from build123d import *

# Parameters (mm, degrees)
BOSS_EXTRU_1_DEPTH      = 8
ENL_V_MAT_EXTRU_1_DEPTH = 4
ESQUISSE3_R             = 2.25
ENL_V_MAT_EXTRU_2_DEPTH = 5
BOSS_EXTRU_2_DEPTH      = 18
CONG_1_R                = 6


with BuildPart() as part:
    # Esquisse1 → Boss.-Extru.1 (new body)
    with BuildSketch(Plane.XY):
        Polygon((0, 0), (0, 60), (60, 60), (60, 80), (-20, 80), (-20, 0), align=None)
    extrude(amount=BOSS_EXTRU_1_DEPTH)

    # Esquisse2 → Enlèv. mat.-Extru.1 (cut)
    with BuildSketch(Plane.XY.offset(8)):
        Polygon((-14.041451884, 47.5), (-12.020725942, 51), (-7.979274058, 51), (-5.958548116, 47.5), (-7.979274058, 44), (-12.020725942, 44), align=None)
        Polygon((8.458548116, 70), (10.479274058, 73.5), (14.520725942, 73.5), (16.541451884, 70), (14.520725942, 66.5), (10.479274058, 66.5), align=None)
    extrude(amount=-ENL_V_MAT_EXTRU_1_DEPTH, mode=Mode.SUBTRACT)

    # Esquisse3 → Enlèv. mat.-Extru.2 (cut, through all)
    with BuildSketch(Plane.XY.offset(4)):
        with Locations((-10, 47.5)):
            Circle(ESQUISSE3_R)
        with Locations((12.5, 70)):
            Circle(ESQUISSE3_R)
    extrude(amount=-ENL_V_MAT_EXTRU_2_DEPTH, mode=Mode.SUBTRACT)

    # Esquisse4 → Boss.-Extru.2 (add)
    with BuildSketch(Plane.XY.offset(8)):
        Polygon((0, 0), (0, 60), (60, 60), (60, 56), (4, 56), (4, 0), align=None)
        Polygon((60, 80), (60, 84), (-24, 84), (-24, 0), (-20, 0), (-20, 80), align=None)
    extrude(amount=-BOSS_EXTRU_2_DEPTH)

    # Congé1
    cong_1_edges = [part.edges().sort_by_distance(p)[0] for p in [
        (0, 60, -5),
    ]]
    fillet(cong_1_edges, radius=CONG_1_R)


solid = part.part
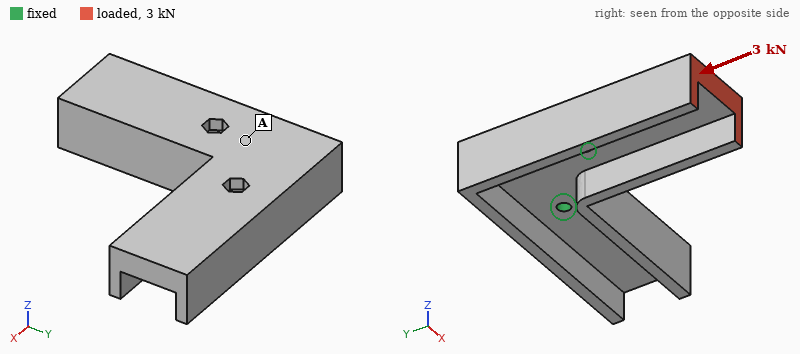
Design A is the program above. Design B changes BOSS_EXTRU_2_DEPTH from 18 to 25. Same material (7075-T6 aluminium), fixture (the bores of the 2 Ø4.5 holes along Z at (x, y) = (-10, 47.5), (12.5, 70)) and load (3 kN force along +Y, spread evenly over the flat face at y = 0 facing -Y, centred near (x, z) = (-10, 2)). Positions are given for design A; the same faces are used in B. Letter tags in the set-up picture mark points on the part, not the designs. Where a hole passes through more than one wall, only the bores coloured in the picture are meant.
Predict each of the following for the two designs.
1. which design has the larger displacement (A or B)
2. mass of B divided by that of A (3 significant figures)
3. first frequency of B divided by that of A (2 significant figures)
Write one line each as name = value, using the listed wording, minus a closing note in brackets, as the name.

which design has the larger displacement = B
mass of B divided by that of A = 1.19
first frequency of B divided by that of A = 0.90
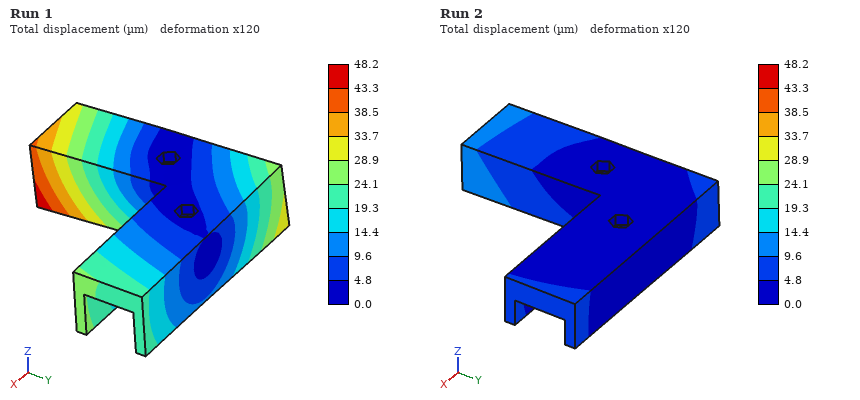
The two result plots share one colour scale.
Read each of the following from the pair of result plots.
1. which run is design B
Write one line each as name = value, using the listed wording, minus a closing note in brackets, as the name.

which run is design B = Run 1
